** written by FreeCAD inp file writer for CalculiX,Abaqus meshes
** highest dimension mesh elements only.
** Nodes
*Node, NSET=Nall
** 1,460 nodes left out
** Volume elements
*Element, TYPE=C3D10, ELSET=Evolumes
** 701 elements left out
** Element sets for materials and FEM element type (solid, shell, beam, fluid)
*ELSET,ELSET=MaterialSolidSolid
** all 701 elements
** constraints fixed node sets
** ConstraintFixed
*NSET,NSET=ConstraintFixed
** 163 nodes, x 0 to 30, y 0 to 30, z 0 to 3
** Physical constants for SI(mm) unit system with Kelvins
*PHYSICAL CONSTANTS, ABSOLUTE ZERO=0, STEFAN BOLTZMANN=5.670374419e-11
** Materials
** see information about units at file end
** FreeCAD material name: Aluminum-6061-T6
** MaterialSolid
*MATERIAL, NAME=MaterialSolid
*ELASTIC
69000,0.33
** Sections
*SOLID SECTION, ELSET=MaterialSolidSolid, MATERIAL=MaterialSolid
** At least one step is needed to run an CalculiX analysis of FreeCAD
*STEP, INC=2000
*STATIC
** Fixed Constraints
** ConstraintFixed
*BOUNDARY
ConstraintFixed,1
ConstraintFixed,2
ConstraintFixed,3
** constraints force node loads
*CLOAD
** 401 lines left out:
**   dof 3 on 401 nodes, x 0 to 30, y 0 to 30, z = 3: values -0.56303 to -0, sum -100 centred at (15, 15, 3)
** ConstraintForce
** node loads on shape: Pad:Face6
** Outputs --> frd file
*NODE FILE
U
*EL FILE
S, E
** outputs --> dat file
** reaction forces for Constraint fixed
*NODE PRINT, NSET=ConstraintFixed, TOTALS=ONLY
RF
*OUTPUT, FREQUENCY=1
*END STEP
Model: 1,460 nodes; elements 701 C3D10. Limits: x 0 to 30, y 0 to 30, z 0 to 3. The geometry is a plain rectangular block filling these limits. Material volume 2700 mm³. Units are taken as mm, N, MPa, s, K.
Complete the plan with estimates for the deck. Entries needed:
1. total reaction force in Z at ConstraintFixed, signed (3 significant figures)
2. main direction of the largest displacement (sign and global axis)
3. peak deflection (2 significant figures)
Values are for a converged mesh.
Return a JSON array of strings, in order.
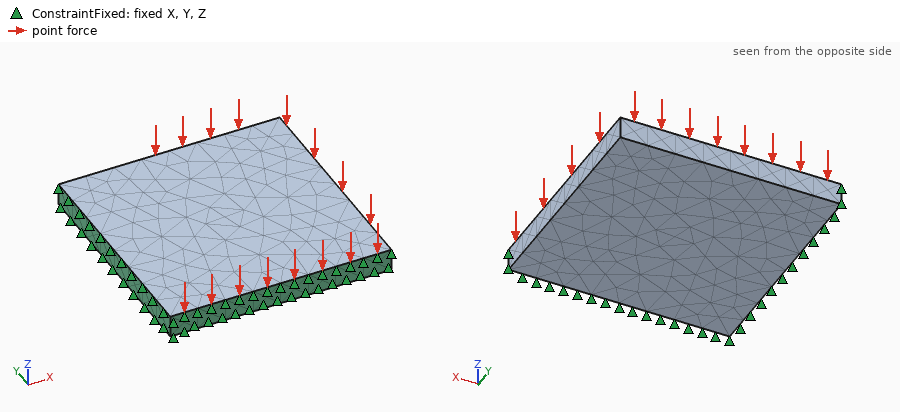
["100 N", "-Z", "0.024 mm"]
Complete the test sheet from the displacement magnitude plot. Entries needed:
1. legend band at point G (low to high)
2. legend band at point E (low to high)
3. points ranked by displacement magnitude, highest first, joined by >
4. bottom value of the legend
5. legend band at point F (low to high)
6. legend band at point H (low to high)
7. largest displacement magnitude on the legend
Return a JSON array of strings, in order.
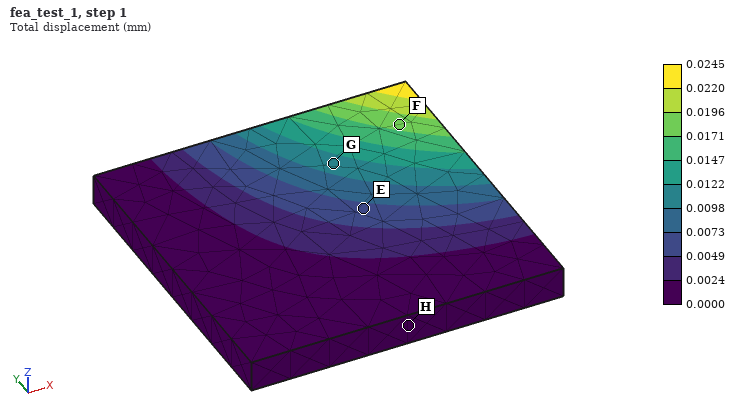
["0.0098 to 0.0122 mm", "0.0049 to 0.0073 mm", "F > G > E > H", "0.0000 mm", "0.0171 to 0.0196 mm", "0.0000 to 0.0024 mm", "0.0245 mm"]
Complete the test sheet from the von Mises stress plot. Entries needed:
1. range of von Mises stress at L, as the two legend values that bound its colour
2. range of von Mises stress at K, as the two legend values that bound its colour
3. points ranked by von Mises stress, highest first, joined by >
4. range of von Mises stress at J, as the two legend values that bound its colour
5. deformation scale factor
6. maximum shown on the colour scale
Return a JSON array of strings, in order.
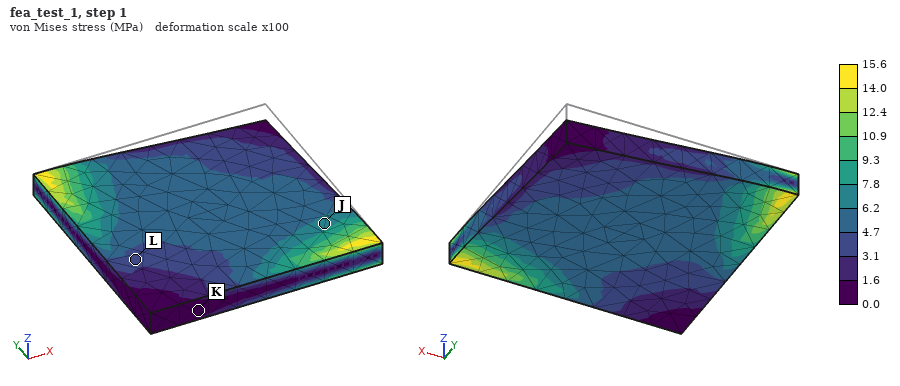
["3.1 to 4.7 MPa", "0.0 to 1.6 MPa", "J > L > K", "6.2 to 7.8 MPa", "100", "15.6 MPa"]
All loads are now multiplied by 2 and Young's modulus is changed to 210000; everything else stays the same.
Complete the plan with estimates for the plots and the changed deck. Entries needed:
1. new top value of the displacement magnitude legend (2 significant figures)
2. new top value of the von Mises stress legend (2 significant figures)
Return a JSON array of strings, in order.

["0.016 mm", "31 MPa"]
